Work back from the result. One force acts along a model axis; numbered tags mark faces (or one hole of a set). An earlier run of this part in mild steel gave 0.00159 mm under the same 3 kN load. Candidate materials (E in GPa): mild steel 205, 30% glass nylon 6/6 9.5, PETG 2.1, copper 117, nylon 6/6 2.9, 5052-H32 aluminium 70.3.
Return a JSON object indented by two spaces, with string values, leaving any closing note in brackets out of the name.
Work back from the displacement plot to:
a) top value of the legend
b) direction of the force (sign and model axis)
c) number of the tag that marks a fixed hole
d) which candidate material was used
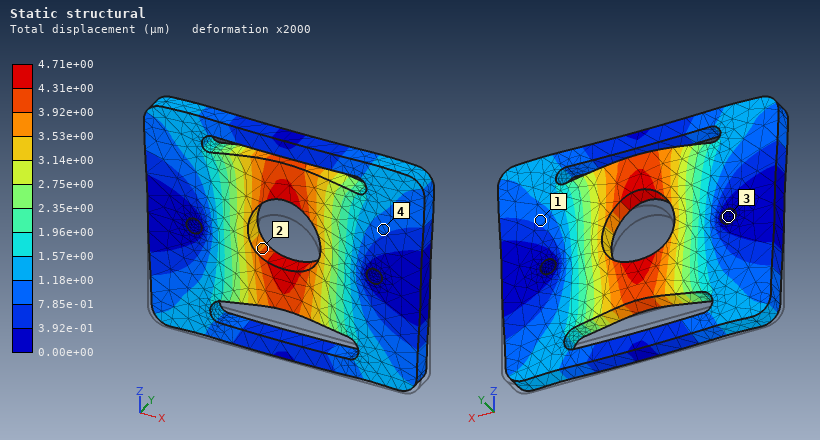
{
  "top value of the legend": "4.71e+00 µm",
  "direction of the force": "+Z",
  "number of the tag that marks a fixed hole": "3",
  "which candidate material was used": "5052-H32 aluminium"
}
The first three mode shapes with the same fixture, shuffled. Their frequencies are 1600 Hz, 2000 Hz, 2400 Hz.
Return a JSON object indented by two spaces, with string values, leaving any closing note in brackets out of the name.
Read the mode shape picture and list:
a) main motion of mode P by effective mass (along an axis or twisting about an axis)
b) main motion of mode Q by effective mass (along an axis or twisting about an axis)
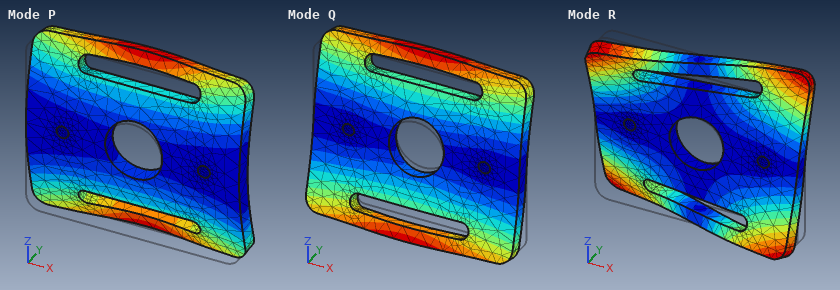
{
  "main motion of mode P by effective mass": "along Y",
  "main motion of mode Q by effective mass": "twisting about X"
}
